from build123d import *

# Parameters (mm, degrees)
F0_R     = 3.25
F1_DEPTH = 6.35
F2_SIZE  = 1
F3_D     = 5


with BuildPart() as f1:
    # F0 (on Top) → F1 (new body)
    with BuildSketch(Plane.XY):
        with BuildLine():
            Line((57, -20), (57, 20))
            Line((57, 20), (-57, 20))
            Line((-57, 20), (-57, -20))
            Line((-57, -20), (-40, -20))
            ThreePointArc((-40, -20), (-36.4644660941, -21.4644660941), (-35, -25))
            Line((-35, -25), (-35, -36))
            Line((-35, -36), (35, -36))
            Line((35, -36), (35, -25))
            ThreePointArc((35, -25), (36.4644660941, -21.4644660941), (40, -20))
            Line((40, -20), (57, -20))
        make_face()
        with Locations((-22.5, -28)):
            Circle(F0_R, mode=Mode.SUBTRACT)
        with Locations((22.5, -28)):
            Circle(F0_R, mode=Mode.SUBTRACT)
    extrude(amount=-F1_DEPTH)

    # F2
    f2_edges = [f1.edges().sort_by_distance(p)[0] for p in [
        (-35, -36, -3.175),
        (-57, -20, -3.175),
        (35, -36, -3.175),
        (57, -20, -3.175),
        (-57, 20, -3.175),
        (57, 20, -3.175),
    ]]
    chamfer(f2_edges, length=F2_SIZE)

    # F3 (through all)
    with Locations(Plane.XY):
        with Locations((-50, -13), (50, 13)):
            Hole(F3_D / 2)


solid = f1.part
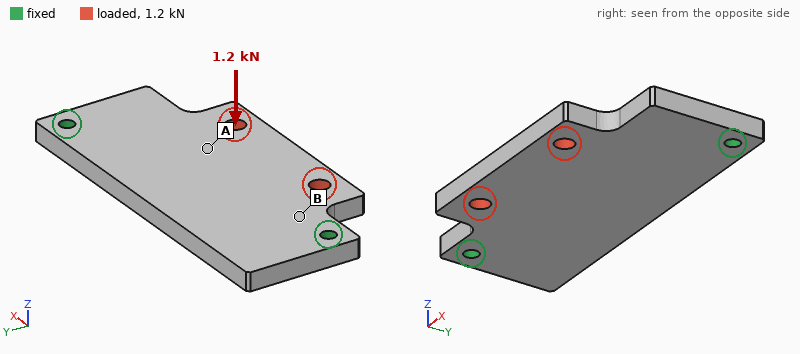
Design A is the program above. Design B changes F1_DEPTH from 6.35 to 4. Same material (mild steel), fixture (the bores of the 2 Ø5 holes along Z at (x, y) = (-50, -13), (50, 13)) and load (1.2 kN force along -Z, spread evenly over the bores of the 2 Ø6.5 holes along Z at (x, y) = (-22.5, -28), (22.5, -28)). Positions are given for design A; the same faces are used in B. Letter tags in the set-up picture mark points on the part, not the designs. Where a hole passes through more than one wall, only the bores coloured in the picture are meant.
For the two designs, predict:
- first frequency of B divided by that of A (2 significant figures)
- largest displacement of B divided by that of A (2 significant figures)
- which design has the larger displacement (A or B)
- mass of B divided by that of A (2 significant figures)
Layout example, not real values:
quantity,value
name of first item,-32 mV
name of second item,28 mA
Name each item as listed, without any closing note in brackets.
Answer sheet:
quantity,value
first frequency of B divided by that of A,0.66
largest displacement of B divided by that of A,3.7
which design has the larger displacement,B
mass of B divided by that of A,0.63
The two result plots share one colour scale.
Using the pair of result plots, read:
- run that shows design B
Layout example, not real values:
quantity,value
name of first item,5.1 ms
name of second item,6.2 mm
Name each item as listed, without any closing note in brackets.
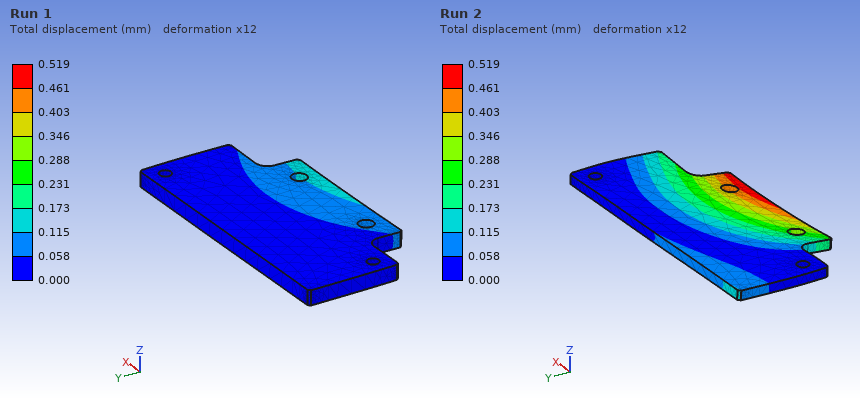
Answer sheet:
quantity,value
run that shows design B,Run 2
